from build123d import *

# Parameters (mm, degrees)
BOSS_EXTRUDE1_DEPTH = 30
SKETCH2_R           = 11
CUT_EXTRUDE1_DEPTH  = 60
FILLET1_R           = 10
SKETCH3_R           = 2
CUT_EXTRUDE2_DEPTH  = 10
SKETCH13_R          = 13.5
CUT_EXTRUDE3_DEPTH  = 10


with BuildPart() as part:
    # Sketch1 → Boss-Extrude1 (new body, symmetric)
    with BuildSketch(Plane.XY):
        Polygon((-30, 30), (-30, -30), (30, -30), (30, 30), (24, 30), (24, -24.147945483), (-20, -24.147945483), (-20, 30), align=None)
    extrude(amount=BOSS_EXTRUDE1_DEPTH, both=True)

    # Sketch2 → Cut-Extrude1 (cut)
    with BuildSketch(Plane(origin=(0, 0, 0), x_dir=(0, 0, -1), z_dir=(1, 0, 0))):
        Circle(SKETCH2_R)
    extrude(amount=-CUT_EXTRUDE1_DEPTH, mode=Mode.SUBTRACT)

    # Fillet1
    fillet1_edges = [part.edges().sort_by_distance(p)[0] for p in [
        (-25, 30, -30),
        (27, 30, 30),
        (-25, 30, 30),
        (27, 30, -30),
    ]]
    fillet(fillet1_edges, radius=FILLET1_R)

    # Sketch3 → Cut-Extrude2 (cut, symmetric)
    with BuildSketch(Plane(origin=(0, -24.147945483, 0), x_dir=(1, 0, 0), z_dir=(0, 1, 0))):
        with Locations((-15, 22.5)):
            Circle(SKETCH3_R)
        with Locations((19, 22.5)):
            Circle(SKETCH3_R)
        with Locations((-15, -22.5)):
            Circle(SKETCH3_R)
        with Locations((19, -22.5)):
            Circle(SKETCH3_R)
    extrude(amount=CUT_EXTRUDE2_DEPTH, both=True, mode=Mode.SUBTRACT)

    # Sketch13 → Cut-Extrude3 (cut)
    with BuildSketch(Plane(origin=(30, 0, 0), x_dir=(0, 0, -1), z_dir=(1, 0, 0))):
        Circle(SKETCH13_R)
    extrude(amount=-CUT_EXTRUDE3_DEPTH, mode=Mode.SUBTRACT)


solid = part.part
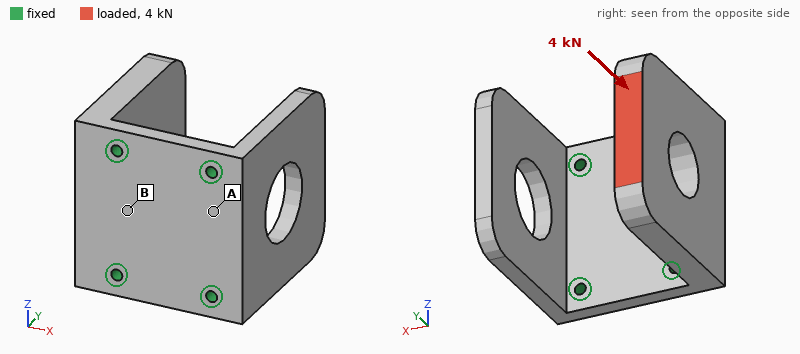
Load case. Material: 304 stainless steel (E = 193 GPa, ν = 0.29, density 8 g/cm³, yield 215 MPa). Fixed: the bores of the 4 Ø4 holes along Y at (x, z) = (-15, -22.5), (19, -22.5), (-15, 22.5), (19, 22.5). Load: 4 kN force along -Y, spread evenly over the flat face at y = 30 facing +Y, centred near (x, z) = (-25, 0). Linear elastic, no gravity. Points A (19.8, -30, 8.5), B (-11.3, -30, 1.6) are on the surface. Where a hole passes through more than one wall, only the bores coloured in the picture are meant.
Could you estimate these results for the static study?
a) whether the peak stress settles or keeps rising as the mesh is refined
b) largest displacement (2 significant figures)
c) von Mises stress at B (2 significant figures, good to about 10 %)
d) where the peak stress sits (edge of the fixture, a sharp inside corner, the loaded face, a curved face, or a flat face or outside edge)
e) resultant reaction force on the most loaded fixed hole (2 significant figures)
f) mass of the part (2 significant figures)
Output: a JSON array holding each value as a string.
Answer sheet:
["keeps rising", "79 µm", "28 MPa", "edge of the fixture", "2.2 kN", "520 g"]
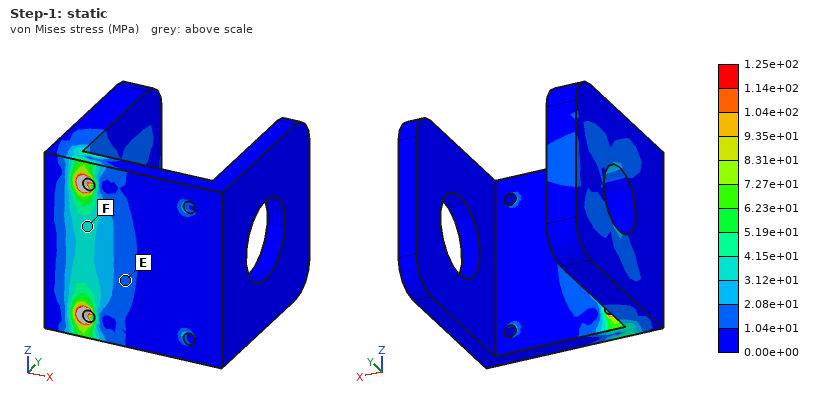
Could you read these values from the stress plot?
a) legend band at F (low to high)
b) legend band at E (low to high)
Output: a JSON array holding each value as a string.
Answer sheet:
["3.12e+01 to 4.15e+01 MPa", "1.04e+01 to 2.08e+01 MPa"]
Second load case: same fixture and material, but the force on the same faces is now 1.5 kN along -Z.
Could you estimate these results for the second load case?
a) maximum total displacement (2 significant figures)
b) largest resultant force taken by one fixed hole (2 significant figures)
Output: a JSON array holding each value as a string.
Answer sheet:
["24 µm", "2.0 kN"]
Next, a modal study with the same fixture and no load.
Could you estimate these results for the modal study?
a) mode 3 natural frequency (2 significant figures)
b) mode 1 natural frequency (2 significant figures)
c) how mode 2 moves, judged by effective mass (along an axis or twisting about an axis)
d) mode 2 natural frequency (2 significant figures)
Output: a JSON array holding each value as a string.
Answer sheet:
["2900 Hz", "1100 Hz", "along X", "1200 Hz"]
